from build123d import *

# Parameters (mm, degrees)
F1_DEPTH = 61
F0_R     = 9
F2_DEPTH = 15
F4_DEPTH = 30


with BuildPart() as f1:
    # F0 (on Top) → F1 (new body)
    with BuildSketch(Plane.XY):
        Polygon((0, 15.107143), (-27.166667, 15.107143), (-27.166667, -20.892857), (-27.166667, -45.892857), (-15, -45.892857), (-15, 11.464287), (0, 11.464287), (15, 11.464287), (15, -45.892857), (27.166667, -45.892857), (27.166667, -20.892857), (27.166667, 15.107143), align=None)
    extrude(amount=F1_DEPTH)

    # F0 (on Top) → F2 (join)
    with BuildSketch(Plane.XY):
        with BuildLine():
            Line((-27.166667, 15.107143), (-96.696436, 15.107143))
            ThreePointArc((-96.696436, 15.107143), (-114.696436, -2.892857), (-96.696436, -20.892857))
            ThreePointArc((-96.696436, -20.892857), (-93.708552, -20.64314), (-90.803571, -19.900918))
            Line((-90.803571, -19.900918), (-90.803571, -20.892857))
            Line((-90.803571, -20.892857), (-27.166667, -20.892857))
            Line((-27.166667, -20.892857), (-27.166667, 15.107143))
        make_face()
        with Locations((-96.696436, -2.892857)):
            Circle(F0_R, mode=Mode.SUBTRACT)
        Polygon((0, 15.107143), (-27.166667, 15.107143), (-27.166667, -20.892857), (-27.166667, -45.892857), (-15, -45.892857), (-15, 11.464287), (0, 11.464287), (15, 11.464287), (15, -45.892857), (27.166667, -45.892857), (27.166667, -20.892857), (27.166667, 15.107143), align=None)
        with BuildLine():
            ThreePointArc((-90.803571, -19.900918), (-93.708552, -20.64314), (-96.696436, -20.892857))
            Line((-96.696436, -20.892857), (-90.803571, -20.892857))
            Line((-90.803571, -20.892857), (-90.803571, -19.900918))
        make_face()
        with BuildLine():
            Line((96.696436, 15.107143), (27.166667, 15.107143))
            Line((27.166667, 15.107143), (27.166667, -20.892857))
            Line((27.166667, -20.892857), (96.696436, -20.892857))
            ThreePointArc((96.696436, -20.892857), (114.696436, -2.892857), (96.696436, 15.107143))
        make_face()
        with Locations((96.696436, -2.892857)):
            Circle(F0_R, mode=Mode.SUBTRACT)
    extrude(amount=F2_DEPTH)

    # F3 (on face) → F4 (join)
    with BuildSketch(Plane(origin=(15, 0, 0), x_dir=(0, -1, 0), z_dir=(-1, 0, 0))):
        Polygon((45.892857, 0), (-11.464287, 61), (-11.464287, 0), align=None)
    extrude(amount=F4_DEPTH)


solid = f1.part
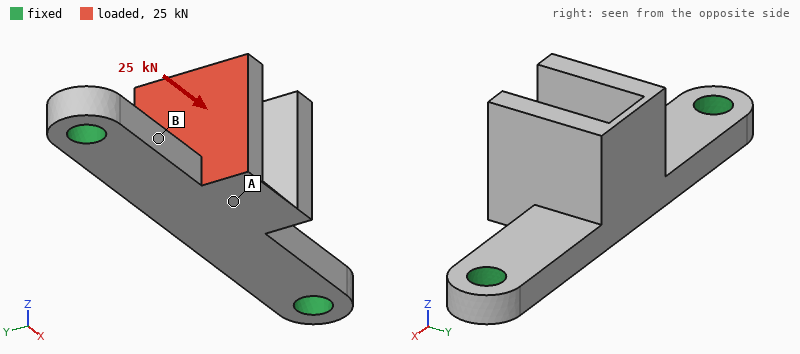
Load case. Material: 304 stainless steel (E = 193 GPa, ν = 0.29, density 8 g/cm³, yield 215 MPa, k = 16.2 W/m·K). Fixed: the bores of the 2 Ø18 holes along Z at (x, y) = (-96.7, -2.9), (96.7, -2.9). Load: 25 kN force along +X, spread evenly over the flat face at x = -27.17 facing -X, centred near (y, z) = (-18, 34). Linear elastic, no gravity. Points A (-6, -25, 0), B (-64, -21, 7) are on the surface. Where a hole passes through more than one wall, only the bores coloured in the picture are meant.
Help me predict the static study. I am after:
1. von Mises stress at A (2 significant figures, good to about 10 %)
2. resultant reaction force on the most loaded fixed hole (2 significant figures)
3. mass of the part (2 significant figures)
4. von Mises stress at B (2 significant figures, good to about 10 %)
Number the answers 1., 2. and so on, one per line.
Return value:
1. 19 MPa
2. 14 kN
3. 1.9 kg
4. 46 MPa
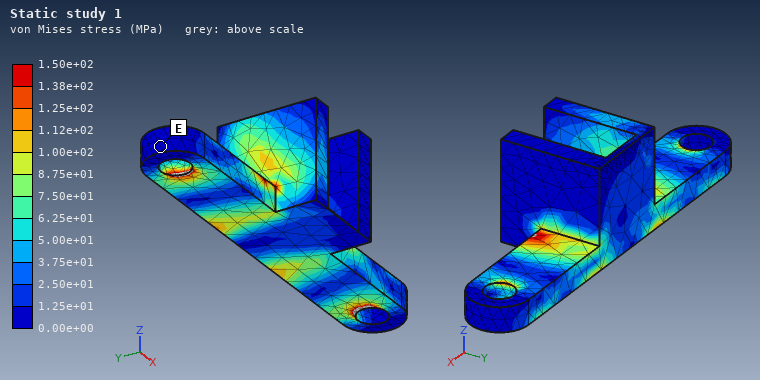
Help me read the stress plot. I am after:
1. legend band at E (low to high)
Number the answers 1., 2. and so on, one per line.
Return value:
1. 0.00e+00 to 1.25e+01 MPa
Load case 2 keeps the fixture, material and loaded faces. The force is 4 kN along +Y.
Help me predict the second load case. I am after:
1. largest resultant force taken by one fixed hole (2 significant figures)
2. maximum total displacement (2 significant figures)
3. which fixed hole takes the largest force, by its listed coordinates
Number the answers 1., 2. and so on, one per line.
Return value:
1. 2.8 kN
2. 0.12 mm
3. (-96.7, -2.9)
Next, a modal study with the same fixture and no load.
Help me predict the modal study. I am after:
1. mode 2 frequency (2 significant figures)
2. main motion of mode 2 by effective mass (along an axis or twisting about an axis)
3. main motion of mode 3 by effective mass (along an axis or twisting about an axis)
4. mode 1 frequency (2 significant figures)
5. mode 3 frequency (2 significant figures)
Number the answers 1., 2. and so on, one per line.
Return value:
1. 1500 Hz
2. along Z
3. along X
4. 1100 Hz
5. 2700 Hz
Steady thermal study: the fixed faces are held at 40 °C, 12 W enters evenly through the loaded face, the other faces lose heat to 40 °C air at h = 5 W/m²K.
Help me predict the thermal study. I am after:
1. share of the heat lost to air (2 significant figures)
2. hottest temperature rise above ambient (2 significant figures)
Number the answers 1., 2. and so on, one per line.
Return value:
1. 36 %
2. 52 K
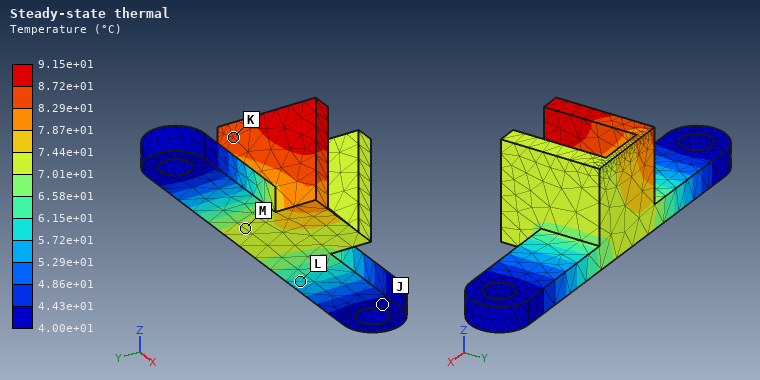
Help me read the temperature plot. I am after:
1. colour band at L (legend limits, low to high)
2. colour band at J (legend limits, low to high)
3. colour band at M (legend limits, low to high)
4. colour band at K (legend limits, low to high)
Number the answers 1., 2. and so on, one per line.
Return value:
1. 5.72e+01 to 6.15e+01 °C
2. 4.00e+01 to 4.43e+01 °C
3. 7.01e+01 to 7.44e+01 °C
4. 8.29e+01 to 8.72e+01 °C
